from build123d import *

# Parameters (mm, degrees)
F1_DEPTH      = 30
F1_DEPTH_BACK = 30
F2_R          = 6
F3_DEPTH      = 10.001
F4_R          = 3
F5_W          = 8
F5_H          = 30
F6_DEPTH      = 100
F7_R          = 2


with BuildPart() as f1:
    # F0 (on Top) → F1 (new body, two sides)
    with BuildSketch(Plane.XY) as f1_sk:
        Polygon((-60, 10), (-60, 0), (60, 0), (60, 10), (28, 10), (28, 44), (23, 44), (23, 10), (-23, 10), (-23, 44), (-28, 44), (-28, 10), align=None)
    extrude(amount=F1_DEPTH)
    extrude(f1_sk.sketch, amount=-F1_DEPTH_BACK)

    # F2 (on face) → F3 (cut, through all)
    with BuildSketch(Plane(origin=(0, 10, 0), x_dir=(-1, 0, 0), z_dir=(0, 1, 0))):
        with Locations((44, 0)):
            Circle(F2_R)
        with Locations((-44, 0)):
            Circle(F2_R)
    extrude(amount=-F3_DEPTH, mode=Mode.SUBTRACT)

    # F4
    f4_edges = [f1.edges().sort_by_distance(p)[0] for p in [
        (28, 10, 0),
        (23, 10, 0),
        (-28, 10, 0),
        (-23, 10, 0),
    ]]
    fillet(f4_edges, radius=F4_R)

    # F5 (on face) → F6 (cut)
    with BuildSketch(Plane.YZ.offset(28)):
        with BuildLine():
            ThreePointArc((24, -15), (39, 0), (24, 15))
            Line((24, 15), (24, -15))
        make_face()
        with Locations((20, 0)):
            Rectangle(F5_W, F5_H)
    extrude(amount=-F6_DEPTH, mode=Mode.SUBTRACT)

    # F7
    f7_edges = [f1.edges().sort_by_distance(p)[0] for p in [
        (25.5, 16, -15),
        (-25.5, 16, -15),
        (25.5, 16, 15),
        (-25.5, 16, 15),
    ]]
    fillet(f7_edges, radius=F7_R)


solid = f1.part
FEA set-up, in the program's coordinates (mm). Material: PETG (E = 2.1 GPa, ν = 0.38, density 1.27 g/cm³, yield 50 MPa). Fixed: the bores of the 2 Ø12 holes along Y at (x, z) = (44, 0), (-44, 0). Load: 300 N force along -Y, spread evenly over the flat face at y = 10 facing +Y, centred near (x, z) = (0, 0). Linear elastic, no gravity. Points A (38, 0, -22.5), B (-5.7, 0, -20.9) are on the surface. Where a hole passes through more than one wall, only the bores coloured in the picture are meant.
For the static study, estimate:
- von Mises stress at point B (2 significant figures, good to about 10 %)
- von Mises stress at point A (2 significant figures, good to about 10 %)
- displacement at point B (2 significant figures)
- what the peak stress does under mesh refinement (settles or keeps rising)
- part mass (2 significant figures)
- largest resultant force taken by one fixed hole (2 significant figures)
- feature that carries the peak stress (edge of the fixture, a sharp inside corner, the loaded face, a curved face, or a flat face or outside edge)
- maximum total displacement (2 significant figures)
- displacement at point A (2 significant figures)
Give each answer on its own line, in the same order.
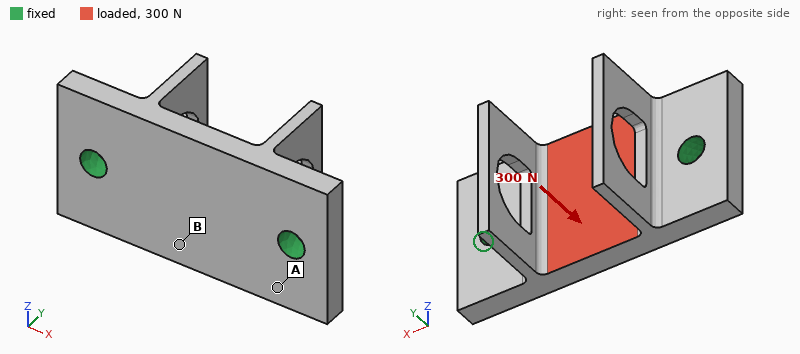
1.8 MPa
0.90 MPa
0.096 mm
keeps rising
110 g
150 N
edge of the fixture
0.13 mm
0.020 mm
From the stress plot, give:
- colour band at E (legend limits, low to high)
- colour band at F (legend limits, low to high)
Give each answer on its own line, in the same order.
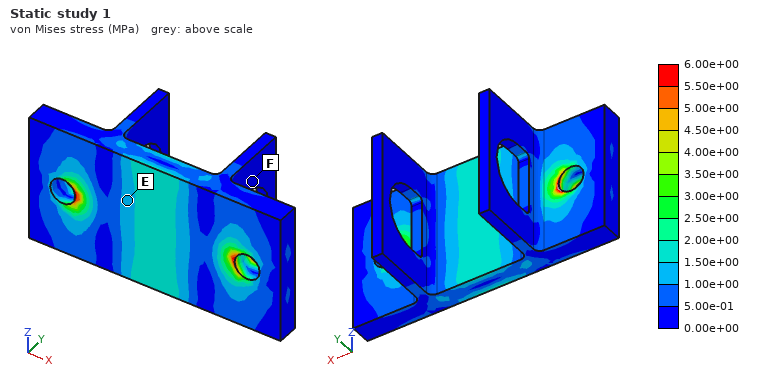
1.00e+00 to 1.50e+00 MPa
0.00e+00 to 5.00e-01 MPa
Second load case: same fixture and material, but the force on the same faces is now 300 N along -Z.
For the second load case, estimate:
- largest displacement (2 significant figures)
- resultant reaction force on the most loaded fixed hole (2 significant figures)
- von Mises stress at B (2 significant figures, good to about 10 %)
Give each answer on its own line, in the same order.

52 µm
150 N
0.71 MPa
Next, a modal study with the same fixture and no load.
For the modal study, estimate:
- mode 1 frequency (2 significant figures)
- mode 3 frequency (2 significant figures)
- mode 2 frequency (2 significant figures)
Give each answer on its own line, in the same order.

680 Hz
1000 Hz
710 Hz
